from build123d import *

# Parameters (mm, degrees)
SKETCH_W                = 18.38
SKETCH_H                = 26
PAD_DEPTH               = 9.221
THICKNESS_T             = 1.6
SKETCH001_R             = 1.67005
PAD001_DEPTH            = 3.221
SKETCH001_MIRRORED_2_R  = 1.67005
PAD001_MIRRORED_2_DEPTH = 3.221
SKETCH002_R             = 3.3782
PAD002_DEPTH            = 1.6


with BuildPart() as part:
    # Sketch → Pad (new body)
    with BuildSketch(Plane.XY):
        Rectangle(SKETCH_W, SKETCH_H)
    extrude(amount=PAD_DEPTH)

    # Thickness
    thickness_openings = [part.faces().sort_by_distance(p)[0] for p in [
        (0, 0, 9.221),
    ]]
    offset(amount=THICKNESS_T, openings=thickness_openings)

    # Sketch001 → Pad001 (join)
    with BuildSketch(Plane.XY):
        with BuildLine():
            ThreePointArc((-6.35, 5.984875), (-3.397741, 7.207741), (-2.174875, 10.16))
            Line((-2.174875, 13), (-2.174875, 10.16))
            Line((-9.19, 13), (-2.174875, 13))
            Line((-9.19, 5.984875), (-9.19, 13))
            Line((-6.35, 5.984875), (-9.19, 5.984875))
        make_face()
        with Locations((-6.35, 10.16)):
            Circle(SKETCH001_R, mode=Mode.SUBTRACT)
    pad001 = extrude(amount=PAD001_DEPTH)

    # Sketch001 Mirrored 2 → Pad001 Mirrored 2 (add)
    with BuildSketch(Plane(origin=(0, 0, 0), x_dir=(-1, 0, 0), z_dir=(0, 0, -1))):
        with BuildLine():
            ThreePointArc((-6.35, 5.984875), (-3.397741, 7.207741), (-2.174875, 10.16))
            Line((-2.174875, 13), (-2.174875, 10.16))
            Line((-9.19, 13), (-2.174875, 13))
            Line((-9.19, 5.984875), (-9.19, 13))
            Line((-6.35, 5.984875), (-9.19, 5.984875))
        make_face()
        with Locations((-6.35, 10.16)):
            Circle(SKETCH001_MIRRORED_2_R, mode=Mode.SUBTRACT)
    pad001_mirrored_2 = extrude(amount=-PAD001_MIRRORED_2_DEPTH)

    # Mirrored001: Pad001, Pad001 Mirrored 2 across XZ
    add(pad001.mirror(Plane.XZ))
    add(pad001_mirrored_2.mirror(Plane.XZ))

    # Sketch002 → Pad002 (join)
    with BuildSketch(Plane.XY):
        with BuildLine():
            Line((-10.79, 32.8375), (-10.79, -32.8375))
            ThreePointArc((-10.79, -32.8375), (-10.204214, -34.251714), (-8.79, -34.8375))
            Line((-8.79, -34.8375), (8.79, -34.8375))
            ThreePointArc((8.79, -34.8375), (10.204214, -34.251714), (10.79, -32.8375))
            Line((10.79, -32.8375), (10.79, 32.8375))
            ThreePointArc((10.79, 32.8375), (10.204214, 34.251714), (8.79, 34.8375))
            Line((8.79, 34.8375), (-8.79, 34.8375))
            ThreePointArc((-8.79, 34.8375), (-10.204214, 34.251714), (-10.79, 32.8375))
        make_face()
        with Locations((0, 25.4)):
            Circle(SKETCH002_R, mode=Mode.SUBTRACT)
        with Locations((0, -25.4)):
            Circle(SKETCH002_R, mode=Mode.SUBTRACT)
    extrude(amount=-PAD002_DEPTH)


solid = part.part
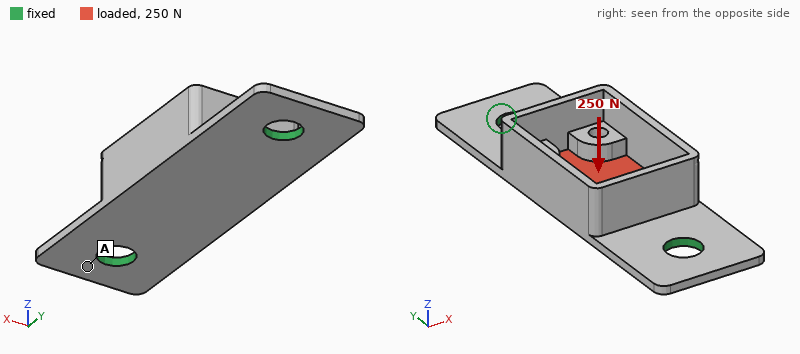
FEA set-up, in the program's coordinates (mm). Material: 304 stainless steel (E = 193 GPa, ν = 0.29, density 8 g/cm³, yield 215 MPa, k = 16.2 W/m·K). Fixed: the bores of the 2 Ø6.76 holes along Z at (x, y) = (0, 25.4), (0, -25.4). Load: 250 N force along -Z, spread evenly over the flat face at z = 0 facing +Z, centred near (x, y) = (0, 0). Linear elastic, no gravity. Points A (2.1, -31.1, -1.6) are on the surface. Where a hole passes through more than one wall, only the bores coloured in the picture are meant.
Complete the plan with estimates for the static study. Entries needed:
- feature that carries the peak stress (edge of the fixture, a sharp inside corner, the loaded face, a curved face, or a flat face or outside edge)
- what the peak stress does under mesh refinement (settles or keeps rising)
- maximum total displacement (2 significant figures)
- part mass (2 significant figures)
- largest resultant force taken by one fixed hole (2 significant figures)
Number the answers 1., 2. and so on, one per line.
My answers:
1. edge of the fixture
2. keeps rising
3. 13 µm
4. 33 g
5. 170 N
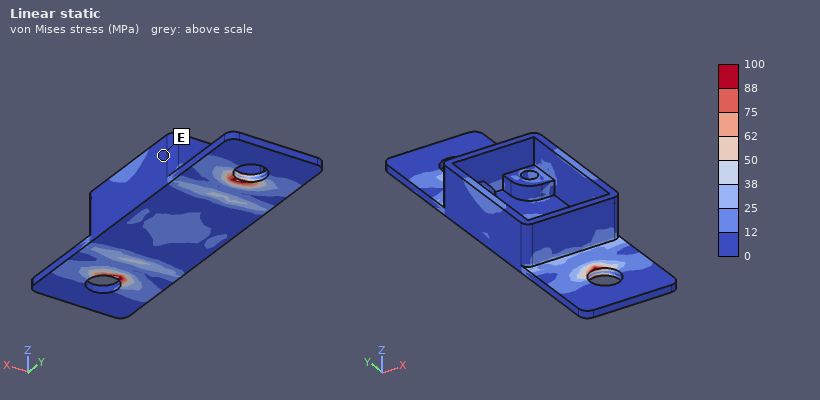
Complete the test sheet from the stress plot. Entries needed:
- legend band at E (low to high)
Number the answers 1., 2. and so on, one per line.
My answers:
1. 0 to 12 MPa
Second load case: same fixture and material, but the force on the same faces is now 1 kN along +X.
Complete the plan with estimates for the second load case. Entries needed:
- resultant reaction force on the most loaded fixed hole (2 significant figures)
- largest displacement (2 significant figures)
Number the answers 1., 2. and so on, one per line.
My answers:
1. 500 N
2. 21 µm
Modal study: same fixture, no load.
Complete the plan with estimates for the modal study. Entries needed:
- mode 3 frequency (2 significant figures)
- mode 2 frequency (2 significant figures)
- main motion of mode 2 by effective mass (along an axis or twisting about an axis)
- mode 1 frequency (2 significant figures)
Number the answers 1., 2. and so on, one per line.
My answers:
1. 9300 Hz
2. 5300 Hz
3. along Z
4. 3500 Hz
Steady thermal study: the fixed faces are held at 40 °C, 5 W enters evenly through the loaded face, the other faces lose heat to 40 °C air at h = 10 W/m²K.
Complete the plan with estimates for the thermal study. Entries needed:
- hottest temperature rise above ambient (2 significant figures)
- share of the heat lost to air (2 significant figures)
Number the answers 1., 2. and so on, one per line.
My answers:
1. 61 K
2. 28 %
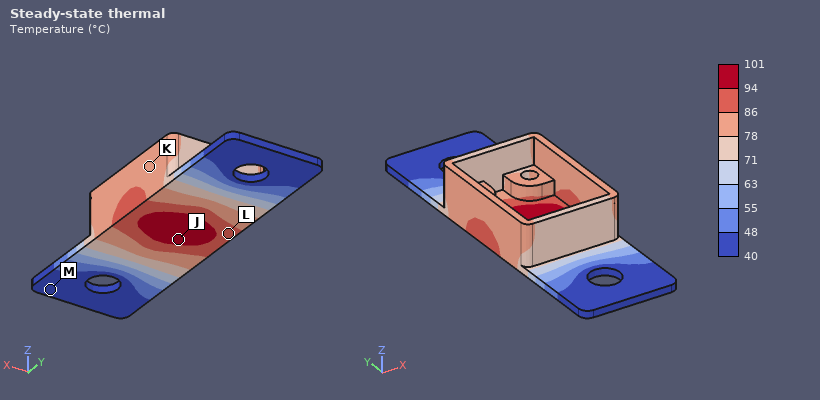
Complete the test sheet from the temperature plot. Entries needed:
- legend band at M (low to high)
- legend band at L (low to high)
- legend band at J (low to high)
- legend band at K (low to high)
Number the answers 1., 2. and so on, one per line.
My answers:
1. 40 to 48 °C
2. 86 to 94 °C
3. 94 to 101 °C
4. 78 to 86 °C
